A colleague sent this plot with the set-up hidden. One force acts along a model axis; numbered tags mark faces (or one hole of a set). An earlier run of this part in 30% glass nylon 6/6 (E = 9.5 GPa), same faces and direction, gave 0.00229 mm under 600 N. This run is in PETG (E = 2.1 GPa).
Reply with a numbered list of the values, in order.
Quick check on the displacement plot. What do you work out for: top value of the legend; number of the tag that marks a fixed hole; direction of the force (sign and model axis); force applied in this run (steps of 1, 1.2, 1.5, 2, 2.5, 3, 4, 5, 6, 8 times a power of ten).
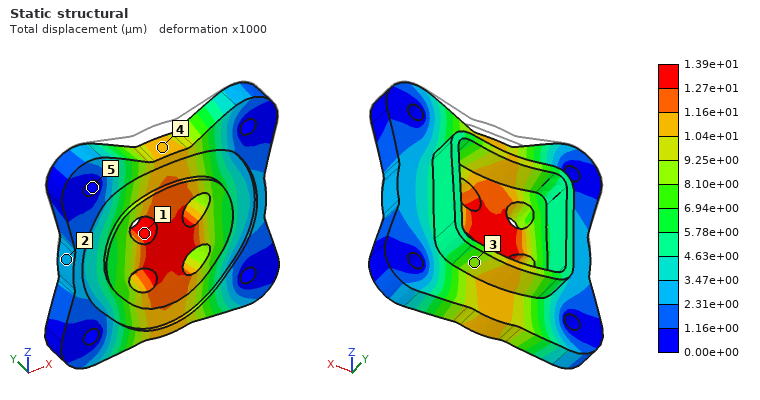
1. 1.39e+01 µm
2. 5
3. -Z
4. 800 N
